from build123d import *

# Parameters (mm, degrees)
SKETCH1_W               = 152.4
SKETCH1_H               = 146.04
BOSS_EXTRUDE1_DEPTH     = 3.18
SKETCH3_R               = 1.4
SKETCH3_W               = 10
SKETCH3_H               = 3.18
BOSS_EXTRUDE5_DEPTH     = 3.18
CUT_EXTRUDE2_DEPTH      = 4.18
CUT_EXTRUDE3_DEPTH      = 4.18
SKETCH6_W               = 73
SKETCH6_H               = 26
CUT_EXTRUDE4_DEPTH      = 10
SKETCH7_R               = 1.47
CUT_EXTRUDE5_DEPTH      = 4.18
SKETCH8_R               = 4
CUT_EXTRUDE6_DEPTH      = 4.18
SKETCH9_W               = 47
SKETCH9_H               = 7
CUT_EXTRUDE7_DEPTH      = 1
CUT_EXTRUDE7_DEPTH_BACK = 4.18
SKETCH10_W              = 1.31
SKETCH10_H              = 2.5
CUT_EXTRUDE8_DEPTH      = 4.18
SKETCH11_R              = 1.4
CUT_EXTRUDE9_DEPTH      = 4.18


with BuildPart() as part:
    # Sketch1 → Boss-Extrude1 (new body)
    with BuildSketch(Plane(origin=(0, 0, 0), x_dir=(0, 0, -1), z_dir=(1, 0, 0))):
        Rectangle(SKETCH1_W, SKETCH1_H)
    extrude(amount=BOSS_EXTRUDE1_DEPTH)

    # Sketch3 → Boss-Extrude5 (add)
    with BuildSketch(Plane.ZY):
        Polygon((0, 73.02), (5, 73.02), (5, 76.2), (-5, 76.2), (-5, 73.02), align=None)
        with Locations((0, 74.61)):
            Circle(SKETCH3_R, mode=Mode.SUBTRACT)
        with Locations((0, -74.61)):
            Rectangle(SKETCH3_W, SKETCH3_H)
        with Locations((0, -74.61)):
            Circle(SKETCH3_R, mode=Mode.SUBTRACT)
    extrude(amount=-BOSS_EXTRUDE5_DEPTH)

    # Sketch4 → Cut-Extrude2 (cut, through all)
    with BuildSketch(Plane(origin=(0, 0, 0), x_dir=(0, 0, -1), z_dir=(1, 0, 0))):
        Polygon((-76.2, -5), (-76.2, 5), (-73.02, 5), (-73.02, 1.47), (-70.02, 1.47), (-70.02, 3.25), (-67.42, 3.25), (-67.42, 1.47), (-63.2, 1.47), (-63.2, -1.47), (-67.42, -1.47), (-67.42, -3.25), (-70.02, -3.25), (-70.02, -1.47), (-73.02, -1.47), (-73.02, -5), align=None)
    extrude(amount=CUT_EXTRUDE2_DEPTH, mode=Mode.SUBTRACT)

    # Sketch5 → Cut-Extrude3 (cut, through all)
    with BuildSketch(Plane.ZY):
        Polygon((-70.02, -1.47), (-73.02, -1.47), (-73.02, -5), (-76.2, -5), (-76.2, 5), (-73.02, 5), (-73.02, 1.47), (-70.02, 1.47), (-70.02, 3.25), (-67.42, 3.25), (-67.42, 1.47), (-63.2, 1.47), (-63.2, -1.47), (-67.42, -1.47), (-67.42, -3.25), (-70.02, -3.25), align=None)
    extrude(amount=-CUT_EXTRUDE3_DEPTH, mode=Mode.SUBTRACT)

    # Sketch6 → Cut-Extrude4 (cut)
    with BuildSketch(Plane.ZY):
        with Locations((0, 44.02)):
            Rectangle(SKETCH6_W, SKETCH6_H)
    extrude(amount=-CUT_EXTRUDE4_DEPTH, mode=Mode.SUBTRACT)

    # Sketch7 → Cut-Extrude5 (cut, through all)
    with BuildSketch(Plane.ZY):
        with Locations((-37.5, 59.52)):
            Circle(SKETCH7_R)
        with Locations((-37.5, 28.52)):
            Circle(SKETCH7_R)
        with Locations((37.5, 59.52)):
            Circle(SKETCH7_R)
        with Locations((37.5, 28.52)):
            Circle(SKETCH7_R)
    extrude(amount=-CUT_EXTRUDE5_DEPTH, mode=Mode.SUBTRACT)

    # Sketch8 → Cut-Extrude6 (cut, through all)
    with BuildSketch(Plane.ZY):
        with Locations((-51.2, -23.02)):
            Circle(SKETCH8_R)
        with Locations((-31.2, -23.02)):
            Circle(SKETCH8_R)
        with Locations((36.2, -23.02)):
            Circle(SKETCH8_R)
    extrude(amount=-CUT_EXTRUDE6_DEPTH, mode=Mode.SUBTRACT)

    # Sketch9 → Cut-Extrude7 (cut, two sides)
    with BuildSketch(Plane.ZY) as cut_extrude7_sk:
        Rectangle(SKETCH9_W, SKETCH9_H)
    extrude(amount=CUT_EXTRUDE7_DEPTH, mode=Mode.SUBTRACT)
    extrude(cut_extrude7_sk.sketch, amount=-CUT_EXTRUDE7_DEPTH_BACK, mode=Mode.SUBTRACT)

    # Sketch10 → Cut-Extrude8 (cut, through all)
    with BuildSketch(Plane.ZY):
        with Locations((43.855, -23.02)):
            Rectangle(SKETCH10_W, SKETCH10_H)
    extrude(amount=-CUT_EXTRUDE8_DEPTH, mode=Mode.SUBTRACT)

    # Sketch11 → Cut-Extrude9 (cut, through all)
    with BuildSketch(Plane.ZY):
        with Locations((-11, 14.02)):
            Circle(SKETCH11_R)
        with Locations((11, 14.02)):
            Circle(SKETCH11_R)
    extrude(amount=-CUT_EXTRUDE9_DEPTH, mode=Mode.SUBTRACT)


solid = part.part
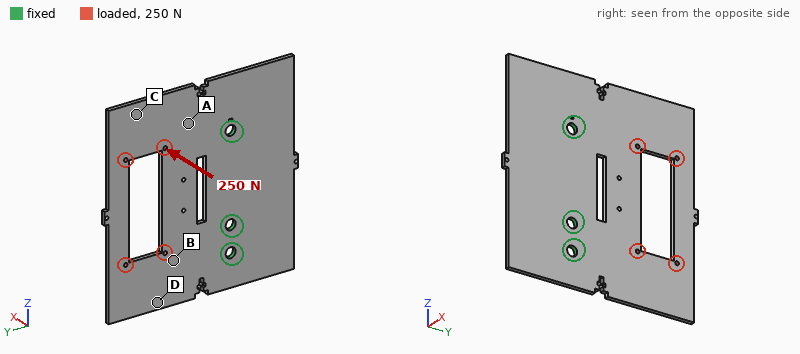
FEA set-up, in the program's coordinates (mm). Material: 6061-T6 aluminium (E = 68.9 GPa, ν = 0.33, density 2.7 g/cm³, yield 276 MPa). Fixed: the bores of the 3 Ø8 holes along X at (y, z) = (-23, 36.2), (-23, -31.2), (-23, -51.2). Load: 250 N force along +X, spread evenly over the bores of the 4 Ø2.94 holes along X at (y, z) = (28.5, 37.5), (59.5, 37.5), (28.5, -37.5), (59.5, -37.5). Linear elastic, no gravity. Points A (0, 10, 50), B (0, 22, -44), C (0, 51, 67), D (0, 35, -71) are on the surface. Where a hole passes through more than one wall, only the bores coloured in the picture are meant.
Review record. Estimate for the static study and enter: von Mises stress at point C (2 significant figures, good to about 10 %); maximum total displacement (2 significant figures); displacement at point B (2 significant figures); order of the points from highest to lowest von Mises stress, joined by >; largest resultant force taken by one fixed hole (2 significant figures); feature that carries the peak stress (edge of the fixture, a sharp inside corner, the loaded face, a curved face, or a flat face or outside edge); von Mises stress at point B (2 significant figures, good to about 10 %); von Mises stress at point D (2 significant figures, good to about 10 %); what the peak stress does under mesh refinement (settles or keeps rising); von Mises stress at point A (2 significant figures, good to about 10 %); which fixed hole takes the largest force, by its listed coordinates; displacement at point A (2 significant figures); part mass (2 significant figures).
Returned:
10 MPa
2.4 mm
0.61 mm
A > B > D > C
120 N
edge of the fixture
35 MPa
22 MPa
keeps rising
48 MPa
(-23, 36.2)
0.40 mm
170 g
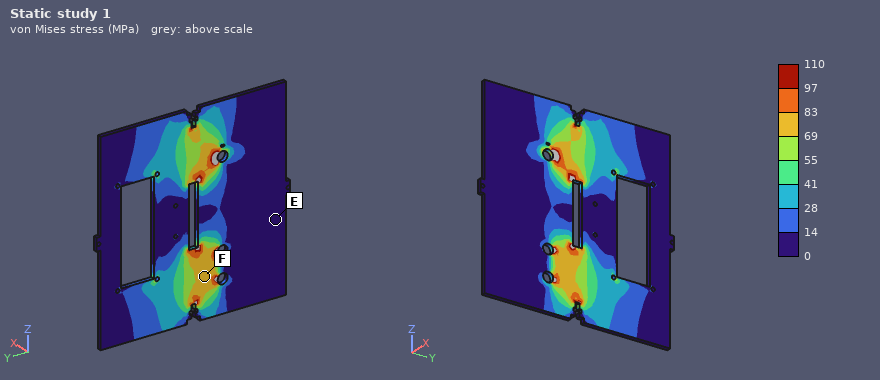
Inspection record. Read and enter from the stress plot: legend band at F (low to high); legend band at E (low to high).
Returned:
69 to 83 MPa
0 to 14 MPa
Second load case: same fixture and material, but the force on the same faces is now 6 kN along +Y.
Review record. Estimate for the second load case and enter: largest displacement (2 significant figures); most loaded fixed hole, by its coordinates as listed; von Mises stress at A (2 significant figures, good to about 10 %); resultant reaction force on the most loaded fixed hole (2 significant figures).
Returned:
55 µm
(-23, 36.2)
27 MPa
3.2 kN
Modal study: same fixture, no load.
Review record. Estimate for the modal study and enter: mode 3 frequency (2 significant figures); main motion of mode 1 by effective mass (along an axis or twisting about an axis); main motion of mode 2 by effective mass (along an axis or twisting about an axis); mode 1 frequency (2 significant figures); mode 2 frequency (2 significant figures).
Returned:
920 Hz
along X
twisting about Y
260 Hz
420 Hz
